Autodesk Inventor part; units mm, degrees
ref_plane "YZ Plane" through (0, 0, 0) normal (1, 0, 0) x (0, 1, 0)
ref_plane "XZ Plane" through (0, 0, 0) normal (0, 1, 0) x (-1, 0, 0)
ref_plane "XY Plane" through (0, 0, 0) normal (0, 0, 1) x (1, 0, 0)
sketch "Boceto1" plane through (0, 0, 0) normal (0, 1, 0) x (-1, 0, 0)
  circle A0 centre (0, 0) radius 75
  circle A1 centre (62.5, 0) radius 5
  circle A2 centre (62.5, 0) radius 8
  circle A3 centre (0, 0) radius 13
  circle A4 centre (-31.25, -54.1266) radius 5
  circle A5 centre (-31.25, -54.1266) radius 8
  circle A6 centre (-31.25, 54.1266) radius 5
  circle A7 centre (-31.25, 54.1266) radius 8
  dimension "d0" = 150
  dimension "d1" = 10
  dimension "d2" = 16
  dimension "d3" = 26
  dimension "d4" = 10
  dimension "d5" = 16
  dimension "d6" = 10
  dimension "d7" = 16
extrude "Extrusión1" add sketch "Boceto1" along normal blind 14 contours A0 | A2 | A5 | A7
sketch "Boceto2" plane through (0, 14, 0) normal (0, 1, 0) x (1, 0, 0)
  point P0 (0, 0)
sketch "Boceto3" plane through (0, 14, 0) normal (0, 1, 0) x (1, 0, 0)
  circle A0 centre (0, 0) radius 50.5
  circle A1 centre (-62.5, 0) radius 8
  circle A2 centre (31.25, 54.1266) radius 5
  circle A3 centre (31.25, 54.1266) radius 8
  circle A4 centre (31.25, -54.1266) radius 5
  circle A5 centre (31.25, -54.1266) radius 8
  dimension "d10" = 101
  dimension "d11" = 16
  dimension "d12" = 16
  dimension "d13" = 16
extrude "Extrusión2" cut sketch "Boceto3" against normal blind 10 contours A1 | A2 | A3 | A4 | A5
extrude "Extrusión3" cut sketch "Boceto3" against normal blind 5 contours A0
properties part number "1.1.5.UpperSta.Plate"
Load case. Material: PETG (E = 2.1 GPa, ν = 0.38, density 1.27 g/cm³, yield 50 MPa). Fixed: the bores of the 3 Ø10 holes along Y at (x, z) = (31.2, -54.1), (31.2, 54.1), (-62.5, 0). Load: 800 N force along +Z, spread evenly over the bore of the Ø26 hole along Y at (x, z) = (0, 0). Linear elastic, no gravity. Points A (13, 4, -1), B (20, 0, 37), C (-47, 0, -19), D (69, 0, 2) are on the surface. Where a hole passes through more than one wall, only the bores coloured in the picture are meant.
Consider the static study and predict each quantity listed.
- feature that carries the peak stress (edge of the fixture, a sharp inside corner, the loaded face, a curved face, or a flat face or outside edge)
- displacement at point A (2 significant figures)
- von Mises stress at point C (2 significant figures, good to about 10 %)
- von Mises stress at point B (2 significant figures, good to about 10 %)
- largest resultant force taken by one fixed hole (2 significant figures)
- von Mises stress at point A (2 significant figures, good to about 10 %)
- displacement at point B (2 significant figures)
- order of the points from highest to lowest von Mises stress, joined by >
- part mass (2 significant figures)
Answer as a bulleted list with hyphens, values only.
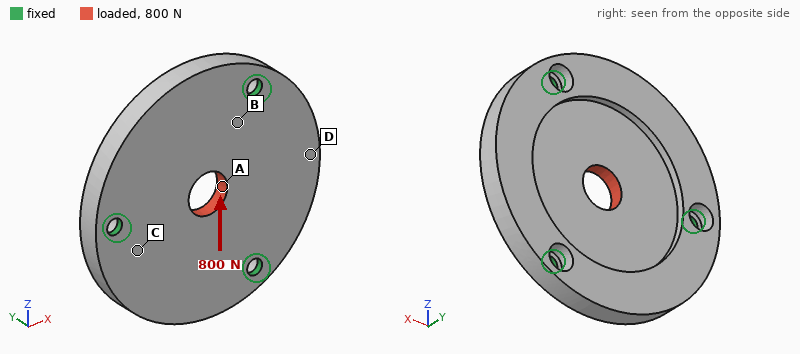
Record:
- edge of the fixture
- 30 µm
- 0.60 MPa
- 1.1 MPa
- 280 N
- 1.9 MPa
- 16 µm
- A > B > C > D
- 250 g
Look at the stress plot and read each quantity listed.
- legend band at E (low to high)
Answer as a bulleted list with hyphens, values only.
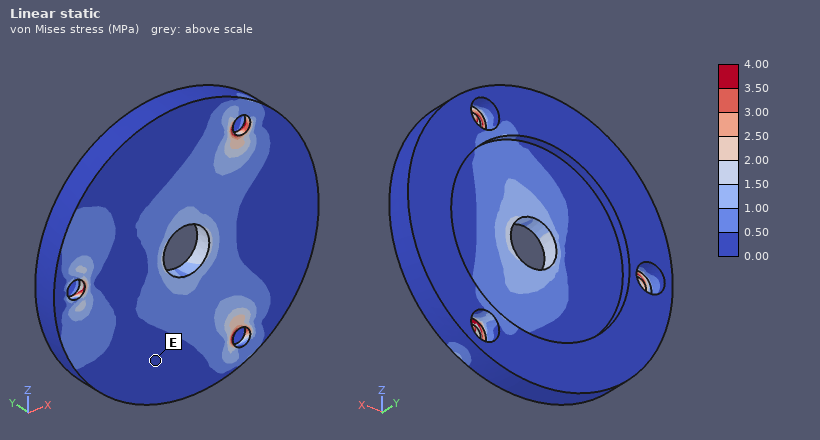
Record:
- 0.00 to 0.50 MPa
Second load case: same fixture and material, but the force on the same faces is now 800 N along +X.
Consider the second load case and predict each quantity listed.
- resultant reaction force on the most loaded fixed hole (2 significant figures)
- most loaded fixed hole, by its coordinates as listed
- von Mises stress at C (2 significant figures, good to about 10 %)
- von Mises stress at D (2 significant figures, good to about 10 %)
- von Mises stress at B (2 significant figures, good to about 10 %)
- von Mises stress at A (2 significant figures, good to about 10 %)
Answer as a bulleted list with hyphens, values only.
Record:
- 290 N
- (-62.5, 0)
- 0.57 MPa
- 0.46 MPa
- 0.71 MPa
- 1.1 MPa
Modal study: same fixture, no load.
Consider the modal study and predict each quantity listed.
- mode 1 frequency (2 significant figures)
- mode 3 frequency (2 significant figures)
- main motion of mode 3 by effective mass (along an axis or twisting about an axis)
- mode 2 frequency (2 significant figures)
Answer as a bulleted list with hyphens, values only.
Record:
- 580 Hz
- 800 Hz
- along Y
- 580 Hz
